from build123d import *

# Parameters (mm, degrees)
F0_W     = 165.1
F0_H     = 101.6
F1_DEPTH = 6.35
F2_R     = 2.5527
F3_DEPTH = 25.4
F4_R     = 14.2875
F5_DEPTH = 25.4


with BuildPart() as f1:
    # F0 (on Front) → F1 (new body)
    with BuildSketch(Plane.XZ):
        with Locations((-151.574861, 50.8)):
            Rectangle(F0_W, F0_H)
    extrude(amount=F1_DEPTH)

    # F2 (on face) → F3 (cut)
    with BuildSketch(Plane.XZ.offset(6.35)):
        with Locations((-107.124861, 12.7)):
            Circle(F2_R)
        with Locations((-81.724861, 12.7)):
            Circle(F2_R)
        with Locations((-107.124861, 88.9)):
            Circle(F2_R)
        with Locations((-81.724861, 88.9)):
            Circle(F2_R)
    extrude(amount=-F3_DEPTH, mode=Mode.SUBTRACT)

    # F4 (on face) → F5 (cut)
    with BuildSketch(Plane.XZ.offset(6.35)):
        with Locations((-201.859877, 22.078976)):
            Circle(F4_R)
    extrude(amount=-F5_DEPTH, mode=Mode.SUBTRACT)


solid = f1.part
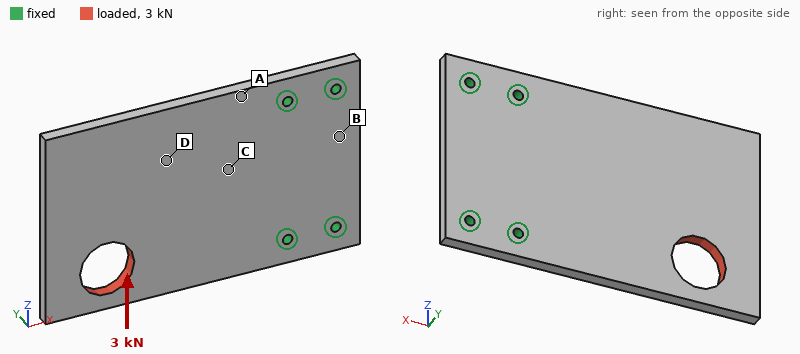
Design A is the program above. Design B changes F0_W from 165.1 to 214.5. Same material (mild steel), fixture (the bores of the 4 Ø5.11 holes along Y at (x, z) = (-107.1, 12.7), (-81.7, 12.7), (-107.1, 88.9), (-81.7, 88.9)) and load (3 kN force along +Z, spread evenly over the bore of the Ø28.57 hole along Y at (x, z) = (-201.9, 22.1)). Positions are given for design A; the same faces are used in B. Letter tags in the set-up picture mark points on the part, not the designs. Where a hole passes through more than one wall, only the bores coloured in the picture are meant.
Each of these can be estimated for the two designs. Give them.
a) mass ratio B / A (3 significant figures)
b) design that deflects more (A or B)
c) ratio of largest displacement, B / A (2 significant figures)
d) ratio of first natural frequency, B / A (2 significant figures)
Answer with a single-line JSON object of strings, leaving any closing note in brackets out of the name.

{"mass ratio B / A": "1.31", "design that deflects more": "B", "ratio of largest displacement, B / A": "1.2", "ratio of first natural frequency, B / A": "0.69"}
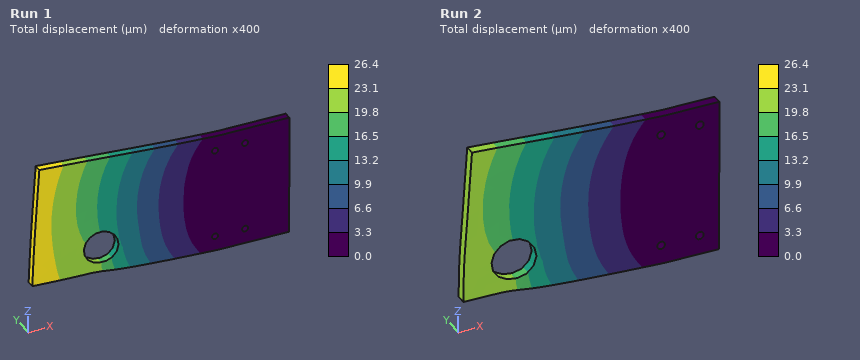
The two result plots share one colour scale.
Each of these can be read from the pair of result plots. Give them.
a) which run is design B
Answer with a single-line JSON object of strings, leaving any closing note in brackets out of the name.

{"which run is design B": "Run 1"}
